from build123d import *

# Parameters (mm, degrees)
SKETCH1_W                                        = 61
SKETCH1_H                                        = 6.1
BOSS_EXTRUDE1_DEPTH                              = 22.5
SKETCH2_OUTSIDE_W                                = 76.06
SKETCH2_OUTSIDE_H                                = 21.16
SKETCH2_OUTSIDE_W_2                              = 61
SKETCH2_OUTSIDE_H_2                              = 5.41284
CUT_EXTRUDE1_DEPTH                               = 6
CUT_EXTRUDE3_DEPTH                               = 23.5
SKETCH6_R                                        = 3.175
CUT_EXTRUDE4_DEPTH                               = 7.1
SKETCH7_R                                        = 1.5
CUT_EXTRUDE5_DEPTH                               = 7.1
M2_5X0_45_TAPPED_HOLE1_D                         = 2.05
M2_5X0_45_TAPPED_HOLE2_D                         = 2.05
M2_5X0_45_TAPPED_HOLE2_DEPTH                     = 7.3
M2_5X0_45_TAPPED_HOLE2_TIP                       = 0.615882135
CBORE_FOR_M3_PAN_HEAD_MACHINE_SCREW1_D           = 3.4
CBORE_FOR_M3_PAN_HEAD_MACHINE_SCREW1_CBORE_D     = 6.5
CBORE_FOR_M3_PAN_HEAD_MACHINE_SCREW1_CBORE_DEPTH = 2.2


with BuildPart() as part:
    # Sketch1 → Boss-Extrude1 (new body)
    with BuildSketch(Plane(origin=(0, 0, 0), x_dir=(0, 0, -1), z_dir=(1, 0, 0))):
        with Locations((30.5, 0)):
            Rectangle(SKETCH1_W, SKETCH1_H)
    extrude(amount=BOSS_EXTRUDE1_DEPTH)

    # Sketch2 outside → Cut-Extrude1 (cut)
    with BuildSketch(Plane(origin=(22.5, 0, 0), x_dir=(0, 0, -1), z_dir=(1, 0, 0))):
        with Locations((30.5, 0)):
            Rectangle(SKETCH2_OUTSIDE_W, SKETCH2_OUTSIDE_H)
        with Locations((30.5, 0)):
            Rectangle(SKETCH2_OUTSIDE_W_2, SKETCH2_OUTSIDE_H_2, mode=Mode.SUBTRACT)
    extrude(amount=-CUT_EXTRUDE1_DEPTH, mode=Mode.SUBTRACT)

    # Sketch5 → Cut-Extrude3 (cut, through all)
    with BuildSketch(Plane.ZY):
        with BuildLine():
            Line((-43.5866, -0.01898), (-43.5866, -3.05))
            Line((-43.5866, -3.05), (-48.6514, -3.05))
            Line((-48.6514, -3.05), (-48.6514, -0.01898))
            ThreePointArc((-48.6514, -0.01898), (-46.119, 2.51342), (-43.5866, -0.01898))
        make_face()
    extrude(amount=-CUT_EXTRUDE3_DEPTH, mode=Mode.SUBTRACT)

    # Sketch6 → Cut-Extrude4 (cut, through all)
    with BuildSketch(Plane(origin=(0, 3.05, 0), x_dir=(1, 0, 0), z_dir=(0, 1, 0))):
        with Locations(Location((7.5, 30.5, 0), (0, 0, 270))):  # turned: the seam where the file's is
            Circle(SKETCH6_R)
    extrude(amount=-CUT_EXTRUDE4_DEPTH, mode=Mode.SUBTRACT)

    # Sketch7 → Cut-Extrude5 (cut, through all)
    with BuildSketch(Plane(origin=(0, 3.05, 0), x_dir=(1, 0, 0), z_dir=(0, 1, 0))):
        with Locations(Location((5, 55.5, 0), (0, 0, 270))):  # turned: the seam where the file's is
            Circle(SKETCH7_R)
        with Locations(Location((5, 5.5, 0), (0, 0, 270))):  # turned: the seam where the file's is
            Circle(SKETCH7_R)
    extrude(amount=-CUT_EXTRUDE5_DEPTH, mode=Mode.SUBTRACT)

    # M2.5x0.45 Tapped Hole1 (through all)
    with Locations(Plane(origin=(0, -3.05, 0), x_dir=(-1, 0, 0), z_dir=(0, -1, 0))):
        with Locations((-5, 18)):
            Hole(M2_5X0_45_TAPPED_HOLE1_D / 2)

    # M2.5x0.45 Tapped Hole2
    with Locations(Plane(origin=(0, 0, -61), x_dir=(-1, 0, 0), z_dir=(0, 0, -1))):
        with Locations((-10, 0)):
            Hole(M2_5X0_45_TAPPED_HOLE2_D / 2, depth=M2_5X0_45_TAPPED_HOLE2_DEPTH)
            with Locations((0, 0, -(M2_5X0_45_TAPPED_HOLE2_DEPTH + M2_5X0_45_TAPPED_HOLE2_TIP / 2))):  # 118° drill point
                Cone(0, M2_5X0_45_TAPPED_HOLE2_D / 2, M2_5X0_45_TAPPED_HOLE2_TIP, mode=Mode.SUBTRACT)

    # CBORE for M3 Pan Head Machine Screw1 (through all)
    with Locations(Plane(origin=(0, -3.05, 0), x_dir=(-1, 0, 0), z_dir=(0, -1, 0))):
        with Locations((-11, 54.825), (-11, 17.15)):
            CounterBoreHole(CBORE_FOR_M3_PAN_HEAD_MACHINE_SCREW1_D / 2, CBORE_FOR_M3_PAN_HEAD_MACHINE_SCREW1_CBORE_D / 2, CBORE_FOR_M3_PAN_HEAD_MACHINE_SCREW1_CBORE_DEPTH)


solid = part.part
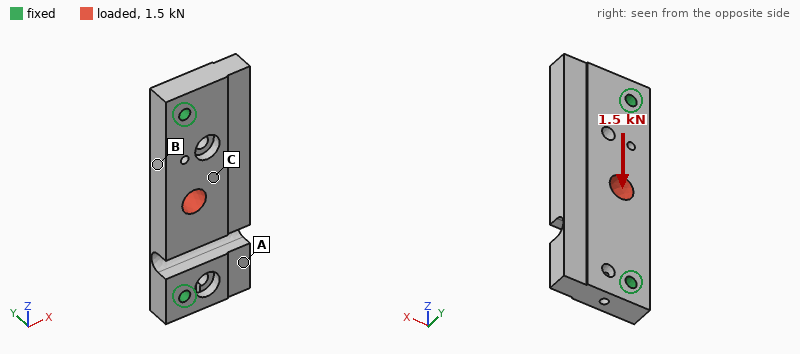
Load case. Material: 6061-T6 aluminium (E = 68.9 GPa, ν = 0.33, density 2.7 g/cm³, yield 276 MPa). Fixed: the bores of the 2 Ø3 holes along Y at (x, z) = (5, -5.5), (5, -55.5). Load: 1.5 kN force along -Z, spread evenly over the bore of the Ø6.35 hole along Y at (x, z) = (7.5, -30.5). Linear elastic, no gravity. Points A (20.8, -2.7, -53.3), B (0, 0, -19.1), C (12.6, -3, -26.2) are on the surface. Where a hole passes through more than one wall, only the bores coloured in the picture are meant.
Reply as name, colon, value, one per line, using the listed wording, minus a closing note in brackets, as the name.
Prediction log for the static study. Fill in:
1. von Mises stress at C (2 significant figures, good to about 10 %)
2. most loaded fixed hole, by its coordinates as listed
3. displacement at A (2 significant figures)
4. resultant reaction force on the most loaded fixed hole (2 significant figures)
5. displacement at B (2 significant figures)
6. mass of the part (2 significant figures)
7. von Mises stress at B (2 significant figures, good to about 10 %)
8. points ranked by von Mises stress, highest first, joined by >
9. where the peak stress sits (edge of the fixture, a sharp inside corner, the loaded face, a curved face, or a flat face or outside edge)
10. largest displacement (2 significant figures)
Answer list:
von Mises stress at C: 11 MPa
most loaded fixed hole, by its coordinates as listed: (5, -5.5)
displacement at A: 1.9 µm
resultant reaction force on the most loaded fixed hole: 1.2 kN
displacement at B: 3.5 µm
mass of the part: 19 g
von Mises stress at B: 19 MPa
points ranked by von Mises stress, highest first, joined by >: B > C > A
where the peak stress sits: a curved face
largest displacement: 10 µm
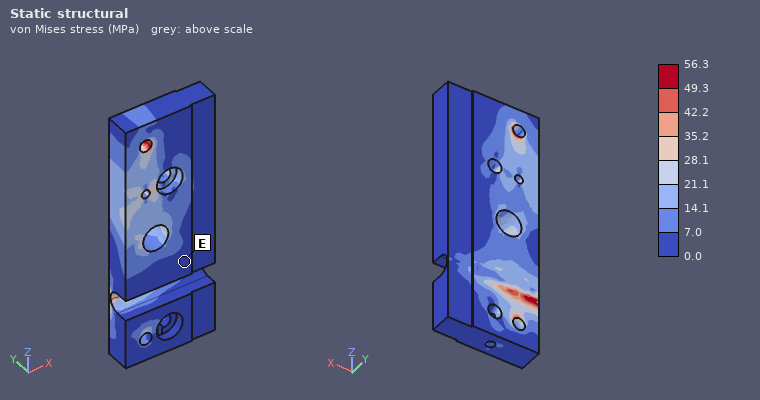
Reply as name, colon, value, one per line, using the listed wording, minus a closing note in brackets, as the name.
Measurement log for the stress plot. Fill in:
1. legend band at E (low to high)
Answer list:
legend band at E: 0.0 to 7.0 MPa
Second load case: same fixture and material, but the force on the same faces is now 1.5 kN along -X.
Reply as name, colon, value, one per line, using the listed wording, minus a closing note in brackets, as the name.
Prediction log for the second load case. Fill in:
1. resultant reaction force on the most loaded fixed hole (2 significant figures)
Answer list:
resultant reaction force on the most loaded fixed hole: 840 N
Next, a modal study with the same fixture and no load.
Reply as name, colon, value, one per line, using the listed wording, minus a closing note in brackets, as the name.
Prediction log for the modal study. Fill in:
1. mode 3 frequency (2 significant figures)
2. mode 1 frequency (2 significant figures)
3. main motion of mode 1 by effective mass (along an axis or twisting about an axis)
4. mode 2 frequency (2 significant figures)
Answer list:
mode 3 frequency: 12 kHz
mode 1 frequency: 6200 Hz
main motion of mode 1 by effective mass: along Y
mode 2 frequency: 9300 Hz
